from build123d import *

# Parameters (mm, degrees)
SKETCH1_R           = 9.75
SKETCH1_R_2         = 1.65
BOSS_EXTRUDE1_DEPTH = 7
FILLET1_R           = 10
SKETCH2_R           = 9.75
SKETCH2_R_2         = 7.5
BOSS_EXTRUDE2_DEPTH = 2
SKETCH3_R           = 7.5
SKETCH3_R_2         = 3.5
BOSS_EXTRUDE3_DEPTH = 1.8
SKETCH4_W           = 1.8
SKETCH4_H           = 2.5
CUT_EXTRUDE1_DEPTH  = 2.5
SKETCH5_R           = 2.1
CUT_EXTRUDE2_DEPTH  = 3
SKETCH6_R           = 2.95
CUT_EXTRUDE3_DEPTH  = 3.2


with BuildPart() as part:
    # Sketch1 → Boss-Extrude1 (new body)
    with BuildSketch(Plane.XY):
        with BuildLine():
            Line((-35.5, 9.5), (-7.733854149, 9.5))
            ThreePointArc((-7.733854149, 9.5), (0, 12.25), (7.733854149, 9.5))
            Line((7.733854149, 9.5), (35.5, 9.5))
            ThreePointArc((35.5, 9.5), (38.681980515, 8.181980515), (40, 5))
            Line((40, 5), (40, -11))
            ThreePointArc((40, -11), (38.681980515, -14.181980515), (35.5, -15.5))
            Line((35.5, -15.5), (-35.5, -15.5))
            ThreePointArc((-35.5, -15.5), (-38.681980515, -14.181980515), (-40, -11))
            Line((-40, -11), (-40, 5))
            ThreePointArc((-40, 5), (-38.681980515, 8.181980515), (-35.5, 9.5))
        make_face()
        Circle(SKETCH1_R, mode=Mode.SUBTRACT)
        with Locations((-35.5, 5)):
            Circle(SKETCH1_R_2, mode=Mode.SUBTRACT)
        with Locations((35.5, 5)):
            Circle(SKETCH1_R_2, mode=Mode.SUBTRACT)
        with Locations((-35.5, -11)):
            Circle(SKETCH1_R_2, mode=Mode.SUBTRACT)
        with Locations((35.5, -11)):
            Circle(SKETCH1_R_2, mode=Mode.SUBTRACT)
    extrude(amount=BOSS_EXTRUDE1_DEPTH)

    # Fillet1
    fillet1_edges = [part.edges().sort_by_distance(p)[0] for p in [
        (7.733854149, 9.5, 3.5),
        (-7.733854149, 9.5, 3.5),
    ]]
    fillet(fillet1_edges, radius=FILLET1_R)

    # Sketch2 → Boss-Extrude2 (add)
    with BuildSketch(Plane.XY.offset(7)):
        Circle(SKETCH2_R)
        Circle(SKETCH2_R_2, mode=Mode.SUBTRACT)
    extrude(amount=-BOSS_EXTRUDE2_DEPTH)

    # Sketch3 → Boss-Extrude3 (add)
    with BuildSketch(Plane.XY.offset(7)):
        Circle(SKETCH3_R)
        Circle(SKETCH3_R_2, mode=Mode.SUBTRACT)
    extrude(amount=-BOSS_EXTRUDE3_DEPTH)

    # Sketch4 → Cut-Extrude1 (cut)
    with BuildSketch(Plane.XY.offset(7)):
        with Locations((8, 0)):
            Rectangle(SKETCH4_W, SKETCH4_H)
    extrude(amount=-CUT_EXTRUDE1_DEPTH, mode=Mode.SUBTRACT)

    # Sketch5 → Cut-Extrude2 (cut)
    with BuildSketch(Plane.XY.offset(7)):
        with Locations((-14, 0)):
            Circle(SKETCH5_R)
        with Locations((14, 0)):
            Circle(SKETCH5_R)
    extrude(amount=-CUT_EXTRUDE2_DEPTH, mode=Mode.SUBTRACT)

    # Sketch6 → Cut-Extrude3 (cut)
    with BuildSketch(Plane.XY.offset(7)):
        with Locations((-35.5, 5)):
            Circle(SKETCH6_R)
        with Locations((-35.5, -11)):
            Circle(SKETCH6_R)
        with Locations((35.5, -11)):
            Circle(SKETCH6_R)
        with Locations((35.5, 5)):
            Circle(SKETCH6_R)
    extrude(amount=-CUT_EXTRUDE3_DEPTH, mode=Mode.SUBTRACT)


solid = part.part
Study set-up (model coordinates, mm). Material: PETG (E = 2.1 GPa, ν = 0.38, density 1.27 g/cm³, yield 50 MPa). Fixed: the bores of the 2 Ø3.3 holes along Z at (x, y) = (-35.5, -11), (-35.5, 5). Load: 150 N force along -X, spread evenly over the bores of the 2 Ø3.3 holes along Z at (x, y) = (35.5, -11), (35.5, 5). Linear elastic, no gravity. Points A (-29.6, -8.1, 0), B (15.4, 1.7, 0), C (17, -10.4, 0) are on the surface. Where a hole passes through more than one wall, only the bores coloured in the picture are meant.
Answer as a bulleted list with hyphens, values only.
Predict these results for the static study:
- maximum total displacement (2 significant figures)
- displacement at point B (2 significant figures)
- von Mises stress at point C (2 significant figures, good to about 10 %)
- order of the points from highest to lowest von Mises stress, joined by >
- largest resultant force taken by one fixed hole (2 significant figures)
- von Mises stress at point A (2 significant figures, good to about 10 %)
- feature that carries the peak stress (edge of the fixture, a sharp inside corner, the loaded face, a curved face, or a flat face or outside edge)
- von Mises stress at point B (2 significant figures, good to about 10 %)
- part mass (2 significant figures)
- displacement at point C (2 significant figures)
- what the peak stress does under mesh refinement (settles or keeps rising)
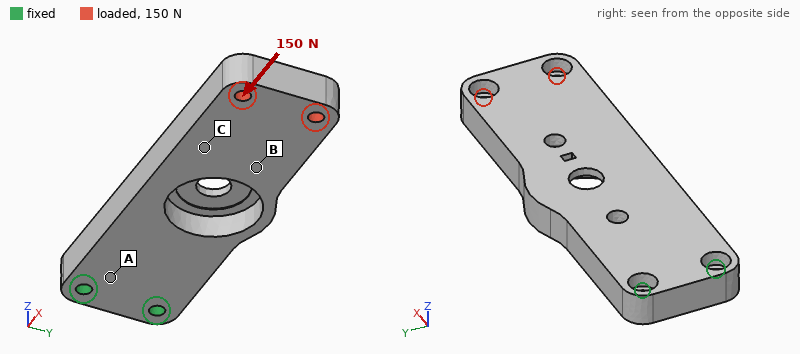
- 0.83 mm
- 0.36 mm
- 2.8 MPa
- C > A > B
- 76 N
- 2.1 MPa
- a sharp inside corner
- 0.90 MPa
- 15 g
- 0.38 mm
- keeps rising
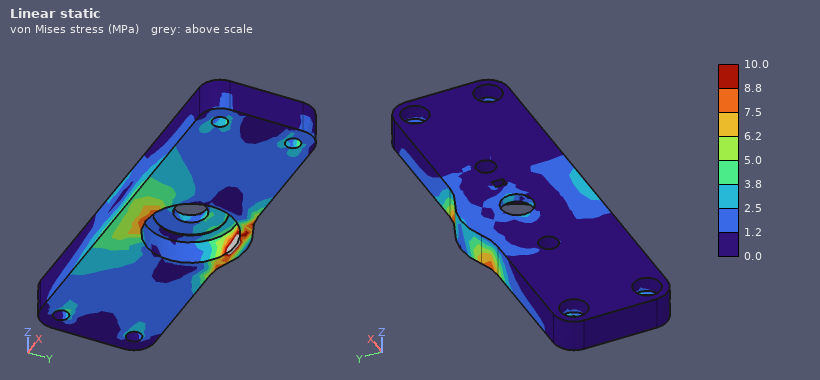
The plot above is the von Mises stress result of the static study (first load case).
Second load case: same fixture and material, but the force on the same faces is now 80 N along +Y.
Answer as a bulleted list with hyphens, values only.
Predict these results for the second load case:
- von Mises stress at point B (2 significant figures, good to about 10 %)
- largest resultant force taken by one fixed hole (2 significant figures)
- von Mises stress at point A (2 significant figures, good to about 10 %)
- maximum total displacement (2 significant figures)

- 1.9 MPa
- 320 N
- 6.4 MPa
- 1.00 mm
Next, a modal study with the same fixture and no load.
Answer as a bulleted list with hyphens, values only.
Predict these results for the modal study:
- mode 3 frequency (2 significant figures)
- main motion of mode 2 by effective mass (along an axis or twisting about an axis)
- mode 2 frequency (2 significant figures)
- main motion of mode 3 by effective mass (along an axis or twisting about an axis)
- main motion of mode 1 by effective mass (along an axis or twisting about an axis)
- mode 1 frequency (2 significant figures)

- 1200 Hz
- along Y
- 730 Hz
- twisting about X
- along Z
- 210 Hz
